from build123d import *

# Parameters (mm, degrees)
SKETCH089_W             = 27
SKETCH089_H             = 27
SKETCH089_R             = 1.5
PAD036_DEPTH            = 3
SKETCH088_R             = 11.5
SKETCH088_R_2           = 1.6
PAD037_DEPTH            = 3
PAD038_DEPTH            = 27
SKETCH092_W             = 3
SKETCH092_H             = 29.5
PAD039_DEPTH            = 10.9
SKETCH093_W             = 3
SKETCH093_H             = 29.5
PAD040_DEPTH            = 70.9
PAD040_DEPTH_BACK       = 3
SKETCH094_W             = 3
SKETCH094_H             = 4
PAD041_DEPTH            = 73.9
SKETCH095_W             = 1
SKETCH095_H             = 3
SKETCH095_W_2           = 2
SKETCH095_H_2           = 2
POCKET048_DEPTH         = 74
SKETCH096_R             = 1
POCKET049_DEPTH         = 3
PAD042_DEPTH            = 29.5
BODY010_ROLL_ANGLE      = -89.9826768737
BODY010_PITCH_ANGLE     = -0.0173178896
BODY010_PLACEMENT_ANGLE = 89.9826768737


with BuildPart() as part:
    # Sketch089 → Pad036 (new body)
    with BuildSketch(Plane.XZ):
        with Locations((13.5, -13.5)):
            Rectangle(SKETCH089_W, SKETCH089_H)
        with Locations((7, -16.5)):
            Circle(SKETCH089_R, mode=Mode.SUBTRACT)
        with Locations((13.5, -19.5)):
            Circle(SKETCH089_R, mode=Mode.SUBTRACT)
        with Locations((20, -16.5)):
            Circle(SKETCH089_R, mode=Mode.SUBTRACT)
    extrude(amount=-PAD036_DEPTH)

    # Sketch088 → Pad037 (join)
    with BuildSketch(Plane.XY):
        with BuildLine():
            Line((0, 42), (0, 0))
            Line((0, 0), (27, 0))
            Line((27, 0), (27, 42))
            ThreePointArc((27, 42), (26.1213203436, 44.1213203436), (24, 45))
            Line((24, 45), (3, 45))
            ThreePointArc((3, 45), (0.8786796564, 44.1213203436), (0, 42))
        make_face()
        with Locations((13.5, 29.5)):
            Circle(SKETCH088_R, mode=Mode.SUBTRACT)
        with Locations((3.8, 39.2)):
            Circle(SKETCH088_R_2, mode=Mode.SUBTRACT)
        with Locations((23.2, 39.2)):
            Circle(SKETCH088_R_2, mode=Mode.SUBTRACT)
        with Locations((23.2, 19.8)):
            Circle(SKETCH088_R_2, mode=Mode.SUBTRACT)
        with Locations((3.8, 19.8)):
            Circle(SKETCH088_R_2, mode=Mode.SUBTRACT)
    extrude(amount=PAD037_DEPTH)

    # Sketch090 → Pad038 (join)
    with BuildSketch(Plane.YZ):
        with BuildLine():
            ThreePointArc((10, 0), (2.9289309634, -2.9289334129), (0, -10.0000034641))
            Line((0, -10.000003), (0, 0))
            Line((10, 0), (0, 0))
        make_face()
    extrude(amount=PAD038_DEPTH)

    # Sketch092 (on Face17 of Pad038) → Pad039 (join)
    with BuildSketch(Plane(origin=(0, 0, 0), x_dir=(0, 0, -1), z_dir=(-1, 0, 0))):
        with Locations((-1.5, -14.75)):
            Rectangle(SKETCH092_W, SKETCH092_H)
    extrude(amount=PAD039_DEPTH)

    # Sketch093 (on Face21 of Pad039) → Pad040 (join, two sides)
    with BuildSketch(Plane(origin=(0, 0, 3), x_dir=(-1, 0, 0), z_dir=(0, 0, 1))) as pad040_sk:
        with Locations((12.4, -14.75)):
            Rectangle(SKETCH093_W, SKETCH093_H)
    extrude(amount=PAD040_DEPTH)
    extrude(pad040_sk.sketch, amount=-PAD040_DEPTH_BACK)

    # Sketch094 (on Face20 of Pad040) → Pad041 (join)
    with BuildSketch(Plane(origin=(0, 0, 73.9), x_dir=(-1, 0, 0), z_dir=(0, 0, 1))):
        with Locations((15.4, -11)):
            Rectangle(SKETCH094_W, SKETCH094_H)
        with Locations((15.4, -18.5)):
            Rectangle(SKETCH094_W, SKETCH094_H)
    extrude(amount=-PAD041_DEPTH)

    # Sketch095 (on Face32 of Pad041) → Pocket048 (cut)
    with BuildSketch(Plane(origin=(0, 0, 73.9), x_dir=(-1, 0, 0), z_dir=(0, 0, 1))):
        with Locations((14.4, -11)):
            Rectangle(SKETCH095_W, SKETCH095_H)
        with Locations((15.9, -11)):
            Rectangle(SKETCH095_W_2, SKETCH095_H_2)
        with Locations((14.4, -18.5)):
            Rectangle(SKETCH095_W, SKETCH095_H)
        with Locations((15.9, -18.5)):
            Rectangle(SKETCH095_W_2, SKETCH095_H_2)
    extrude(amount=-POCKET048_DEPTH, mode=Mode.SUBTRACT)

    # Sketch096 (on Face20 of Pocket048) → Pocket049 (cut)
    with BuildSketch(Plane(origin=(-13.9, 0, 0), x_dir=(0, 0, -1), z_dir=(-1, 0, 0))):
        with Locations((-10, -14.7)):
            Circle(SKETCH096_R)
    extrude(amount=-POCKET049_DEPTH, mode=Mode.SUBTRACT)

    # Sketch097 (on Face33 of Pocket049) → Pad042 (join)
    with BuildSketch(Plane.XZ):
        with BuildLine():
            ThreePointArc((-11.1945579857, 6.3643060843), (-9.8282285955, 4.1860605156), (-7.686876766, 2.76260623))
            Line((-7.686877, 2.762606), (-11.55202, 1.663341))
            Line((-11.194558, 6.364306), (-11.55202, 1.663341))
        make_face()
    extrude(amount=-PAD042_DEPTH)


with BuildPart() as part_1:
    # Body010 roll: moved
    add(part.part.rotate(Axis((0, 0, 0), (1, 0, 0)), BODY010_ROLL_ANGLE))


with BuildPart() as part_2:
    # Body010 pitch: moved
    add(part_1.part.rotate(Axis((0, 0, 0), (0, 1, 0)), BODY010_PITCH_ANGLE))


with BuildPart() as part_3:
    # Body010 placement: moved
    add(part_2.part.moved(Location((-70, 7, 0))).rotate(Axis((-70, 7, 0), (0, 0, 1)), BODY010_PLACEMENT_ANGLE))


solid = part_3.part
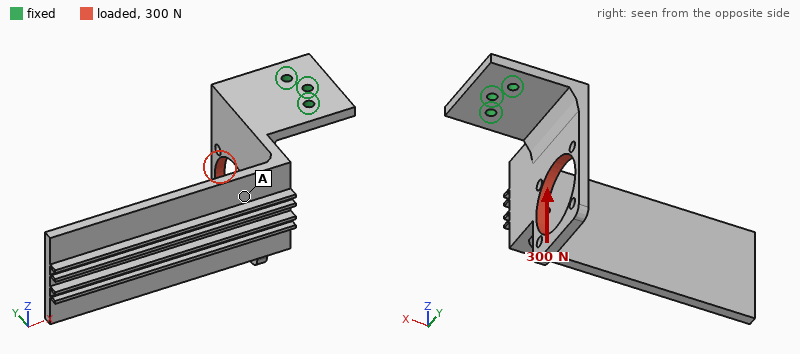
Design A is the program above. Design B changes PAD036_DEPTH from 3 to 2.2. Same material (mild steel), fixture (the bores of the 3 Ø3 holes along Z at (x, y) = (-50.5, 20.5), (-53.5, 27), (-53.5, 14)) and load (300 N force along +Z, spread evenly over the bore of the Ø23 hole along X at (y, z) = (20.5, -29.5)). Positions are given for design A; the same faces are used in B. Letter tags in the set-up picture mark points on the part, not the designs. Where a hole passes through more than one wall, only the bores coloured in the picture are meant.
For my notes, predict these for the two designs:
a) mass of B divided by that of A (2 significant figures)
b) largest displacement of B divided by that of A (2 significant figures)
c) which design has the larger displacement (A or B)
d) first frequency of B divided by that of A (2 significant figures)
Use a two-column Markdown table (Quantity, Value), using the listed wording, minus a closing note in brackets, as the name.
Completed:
| Quantity | Value |
|---|---|
| mass of B divided by that of A | 0.96 |
| largest displacement of B divided by that of A | 2.4 |
| which design has the larger displacement | B |
| first frequency of B divided by that of A | 0.74 |
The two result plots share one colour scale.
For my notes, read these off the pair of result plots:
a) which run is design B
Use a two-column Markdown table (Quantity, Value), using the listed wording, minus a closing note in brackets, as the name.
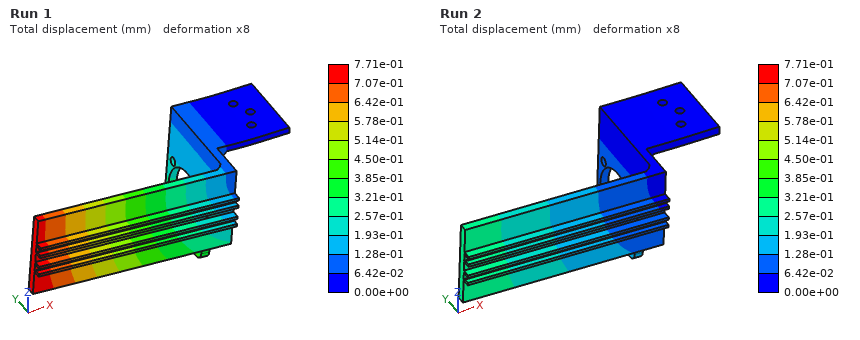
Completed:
| Quantity | Value |
|---|---|
| which run is design B | Run 1 |
